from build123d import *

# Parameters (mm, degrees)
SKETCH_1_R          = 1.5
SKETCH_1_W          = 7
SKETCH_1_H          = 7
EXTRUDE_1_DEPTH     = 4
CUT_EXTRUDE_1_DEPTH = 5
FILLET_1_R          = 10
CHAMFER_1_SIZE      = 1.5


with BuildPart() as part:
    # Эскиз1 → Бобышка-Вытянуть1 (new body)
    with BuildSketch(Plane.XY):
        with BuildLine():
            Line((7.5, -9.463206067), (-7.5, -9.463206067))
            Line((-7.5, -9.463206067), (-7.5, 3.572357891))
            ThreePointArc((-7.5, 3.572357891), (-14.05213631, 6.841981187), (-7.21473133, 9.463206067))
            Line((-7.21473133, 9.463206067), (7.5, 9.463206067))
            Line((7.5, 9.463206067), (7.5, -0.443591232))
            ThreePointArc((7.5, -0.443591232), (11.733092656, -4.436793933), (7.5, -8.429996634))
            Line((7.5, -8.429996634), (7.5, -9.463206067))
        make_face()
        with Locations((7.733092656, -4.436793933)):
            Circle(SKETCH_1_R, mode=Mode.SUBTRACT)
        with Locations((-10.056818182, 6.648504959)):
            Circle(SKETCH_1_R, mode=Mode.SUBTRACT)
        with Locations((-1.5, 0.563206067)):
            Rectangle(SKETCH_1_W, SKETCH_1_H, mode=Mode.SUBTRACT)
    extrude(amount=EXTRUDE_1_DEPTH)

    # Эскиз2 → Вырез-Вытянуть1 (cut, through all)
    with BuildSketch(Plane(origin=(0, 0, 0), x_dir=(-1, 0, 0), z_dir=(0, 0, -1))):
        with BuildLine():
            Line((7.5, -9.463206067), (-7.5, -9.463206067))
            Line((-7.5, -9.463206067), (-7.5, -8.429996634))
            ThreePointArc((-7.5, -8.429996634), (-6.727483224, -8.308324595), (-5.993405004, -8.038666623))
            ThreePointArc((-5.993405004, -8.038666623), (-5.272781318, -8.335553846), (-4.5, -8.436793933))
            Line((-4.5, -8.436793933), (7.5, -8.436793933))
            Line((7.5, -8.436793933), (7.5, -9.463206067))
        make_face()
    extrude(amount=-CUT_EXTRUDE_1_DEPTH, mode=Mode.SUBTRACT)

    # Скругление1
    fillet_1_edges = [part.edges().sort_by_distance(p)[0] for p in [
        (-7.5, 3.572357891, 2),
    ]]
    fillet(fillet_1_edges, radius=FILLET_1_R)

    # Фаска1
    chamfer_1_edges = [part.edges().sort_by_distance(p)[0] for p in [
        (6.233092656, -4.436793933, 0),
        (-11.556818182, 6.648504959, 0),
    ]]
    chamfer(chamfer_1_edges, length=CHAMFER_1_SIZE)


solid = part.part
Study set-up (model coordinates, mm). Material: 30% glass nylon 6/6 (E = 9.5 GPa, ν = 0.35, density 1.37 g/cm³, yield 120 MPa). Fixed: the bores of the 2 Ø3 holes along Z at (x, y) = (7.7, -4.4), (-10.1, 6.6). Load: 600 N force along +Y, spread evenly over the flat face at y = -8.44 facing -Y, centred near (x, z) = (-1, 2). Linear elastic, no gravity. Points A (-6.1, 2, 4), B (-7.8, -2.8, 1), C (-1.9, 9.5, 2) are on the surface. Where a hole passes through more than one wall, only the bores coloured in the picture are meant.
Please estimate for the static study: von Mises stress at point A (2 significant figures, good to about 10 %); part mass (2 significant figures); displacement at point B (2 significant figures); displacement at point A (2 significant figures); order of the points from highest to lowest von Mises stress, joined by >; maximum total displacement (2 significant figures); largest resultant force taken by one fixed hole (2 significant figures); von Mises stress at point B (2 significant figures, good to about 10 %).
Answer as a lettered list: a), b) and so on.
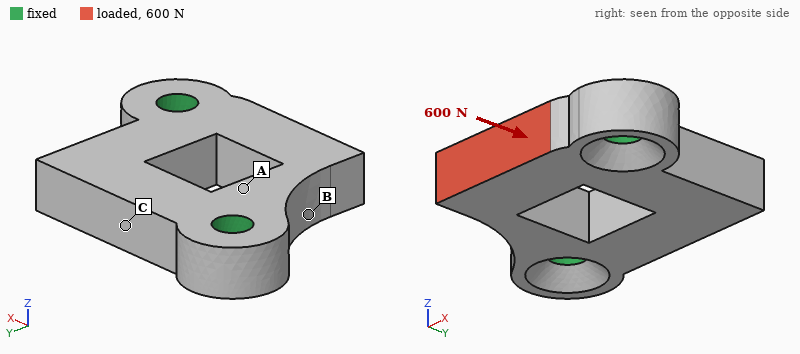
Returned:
a) 16 MPa
b) 1.5 g
c) 27 µm
d) 11 µm
e) B > A > C
f) 43 µm
g) 310 N
h) 26 MPa
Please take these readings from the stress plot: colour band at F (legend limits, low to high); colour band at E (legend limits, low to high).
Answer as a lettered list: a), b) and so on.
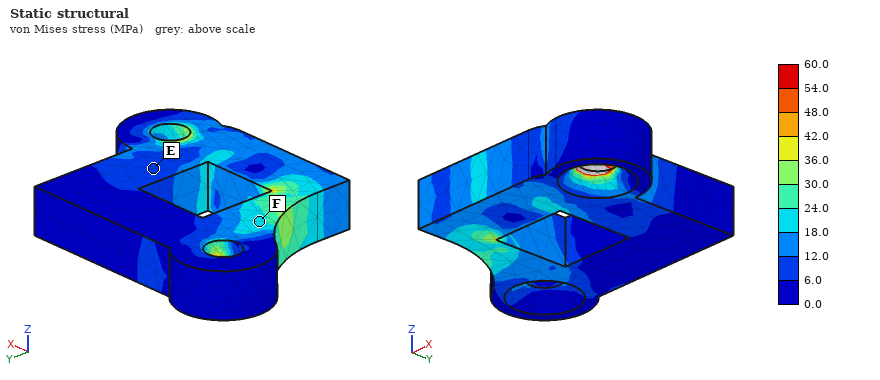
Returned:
a) 18.0 to 24.0 MPa
b) 6.0 to 12.0 MPa
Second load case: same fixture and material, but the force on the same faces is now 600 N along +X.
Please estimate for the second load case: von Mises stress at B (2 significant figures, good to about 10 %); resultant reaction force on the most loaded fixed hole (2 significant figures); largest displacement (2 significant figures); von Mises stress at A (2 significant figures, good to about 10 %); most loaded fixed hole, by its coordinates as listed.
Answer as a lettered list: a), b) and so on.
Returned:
a) 22 MPa
b) 560 N
c) 52 µm
d) 9.9 MPa
e) (7.7, -4.4)
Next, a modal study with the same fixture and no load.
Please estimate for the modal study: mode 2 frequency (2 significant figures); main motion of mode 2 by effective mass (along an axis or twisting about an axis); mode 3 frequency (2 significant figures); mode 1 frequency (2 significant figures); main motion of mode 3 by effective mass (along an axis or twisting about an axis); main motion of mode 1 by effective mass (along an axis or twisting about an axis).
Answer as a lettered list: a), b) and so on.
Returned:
a) 12 kHz
b) along Z
c) 28 kHz
d) 9500 Hz
e) along Y
f) twisting about X
